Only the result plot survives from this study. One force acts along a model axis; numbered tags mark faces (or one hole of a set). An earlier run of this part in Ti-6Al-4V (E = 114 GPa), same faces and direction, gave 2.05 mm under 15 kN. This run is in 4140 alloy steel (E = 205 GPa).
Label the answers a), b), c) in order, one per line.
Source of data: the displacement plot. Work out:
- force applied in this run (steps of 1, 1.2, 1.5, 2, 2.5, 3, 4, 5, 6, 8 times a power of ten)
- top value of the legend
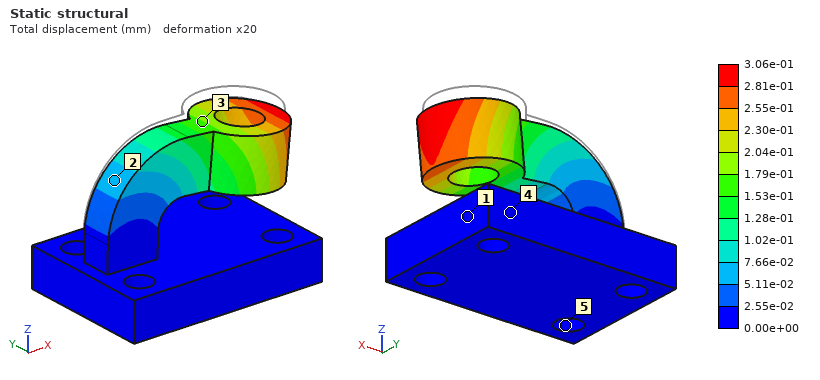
a) 4 kN
b) 3.06e-01 mm
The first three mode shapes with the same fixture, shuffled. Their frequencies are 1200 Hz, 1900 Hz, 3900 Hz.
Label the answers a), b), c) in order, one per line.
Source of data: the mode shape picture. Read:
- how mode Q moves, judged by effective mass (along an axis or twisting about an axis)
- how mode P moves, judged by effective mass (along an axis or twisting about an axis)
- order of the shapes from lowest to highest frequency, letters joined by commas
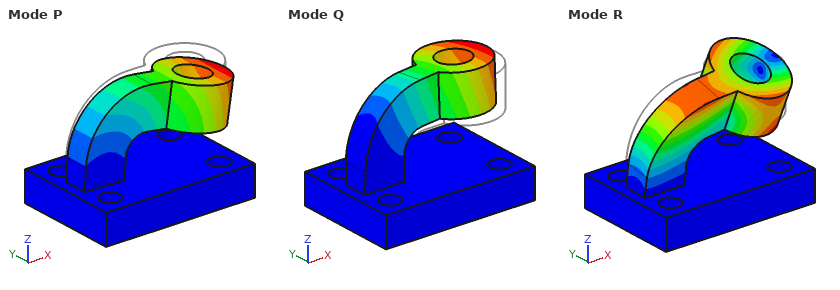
a) along Y
b) along Z
c) Q, P, R
